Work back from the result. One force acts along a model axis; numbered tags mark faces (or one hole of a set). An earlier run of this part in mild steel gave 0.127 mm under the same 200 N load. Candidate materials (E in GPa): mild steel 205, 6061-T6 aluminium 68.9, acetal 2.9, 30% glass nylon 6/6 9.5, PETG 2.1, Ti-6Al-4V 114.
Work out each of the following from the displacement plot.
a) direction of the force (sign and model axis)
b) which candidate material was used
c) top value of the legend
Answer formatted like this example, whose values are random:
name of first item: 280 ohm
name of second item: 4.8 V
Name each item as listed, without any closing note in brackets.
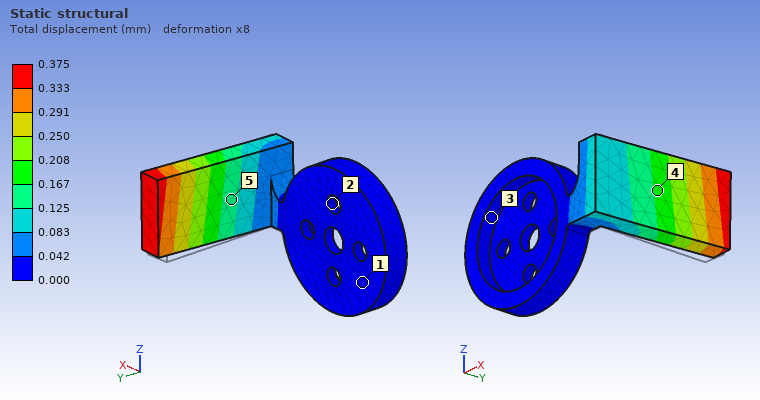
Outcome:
direction of the force: +X
which candidate material was used: 6061-T6 aluminium
top value of the legend: 0.375 mm
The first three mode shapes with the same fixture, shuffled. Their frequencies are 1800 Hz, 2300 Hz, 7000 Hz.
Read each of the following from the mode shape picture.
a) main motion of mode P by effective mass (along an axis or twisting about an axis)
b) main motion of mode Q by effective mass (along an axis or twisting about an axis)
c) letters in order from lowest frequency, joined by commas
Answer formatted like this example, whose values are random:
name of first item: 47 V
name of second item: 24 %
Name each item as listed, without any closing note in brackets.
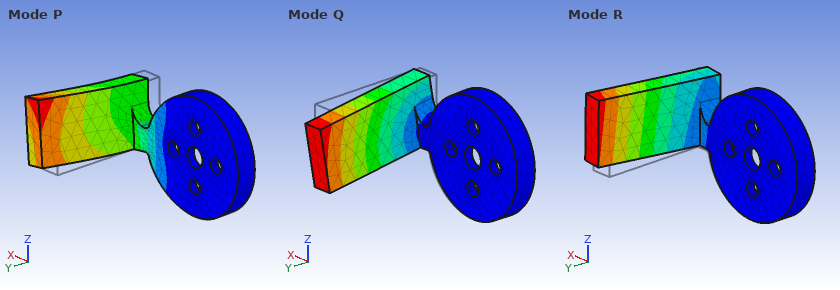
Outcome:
main motion of mode P by effective mass: along Y
main motion of mode Q by effective mass: along Z
letters in order from lowest frequency, joined by commas: R, Q, P
